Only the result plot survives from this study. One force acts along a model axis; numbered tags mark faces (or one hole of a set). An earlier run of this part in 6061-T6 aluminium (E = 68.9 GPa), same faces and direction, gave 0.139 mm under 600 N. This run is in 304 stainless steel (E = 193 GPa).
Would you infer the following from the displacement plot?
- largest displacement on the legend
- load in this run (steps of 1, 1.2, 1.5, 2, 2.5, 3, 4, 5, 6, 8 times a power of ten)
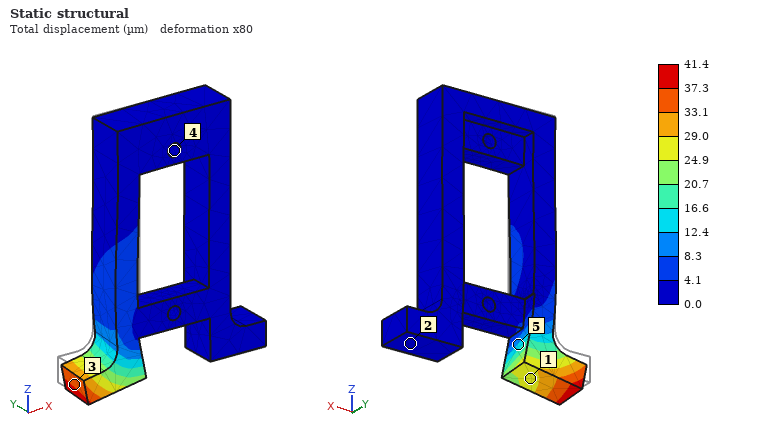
41.4 µm
500 N
